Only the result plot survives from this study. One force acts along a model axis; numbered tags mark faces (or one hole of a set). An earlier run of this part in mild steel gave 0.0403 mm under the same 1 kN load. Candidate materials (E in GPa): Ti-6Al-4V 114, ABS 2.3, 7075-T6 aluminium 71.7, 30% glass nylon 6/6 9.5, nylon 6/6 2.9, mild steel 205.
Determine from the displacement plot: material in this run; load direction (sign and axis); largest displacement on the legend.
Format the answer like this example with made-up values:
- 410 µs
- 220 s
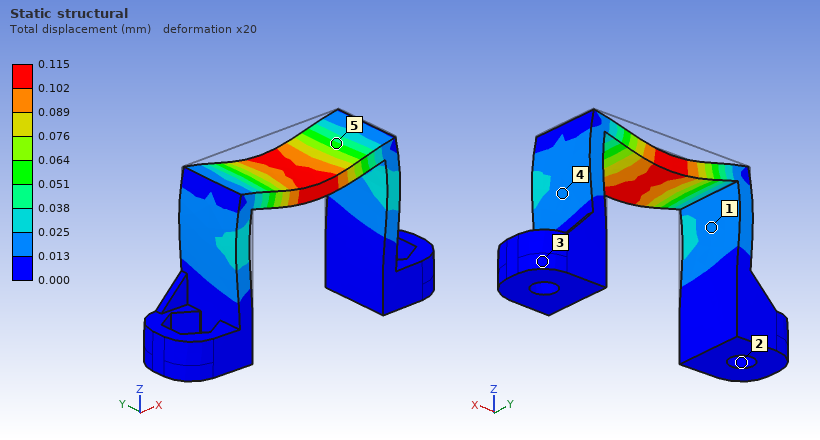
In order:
- 7075-T6 aluminium
- -Z
- 0.115 mm
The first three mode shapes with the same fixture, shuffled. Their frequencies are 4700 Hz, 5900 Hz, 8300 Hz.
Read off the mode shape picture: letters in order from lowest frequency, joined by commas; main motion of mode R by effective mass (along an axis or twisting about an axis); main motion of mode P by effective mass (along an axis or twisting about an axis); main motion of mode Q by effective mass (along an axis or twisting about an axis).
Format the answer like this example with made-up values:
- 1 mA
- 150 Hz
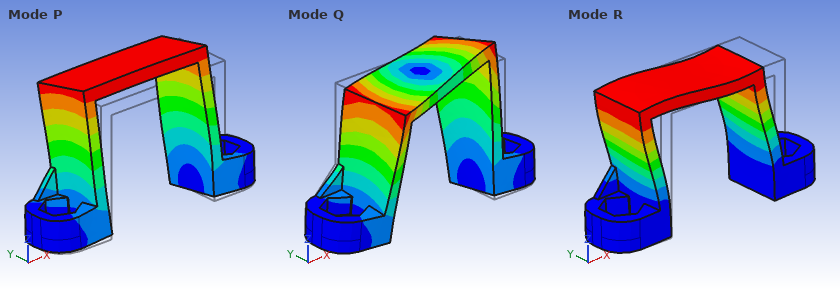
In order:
- R, P, Q
- along X
- along Y
- twisting about Z
